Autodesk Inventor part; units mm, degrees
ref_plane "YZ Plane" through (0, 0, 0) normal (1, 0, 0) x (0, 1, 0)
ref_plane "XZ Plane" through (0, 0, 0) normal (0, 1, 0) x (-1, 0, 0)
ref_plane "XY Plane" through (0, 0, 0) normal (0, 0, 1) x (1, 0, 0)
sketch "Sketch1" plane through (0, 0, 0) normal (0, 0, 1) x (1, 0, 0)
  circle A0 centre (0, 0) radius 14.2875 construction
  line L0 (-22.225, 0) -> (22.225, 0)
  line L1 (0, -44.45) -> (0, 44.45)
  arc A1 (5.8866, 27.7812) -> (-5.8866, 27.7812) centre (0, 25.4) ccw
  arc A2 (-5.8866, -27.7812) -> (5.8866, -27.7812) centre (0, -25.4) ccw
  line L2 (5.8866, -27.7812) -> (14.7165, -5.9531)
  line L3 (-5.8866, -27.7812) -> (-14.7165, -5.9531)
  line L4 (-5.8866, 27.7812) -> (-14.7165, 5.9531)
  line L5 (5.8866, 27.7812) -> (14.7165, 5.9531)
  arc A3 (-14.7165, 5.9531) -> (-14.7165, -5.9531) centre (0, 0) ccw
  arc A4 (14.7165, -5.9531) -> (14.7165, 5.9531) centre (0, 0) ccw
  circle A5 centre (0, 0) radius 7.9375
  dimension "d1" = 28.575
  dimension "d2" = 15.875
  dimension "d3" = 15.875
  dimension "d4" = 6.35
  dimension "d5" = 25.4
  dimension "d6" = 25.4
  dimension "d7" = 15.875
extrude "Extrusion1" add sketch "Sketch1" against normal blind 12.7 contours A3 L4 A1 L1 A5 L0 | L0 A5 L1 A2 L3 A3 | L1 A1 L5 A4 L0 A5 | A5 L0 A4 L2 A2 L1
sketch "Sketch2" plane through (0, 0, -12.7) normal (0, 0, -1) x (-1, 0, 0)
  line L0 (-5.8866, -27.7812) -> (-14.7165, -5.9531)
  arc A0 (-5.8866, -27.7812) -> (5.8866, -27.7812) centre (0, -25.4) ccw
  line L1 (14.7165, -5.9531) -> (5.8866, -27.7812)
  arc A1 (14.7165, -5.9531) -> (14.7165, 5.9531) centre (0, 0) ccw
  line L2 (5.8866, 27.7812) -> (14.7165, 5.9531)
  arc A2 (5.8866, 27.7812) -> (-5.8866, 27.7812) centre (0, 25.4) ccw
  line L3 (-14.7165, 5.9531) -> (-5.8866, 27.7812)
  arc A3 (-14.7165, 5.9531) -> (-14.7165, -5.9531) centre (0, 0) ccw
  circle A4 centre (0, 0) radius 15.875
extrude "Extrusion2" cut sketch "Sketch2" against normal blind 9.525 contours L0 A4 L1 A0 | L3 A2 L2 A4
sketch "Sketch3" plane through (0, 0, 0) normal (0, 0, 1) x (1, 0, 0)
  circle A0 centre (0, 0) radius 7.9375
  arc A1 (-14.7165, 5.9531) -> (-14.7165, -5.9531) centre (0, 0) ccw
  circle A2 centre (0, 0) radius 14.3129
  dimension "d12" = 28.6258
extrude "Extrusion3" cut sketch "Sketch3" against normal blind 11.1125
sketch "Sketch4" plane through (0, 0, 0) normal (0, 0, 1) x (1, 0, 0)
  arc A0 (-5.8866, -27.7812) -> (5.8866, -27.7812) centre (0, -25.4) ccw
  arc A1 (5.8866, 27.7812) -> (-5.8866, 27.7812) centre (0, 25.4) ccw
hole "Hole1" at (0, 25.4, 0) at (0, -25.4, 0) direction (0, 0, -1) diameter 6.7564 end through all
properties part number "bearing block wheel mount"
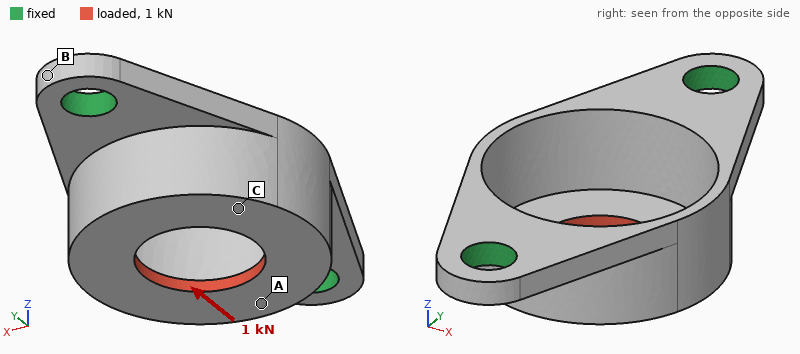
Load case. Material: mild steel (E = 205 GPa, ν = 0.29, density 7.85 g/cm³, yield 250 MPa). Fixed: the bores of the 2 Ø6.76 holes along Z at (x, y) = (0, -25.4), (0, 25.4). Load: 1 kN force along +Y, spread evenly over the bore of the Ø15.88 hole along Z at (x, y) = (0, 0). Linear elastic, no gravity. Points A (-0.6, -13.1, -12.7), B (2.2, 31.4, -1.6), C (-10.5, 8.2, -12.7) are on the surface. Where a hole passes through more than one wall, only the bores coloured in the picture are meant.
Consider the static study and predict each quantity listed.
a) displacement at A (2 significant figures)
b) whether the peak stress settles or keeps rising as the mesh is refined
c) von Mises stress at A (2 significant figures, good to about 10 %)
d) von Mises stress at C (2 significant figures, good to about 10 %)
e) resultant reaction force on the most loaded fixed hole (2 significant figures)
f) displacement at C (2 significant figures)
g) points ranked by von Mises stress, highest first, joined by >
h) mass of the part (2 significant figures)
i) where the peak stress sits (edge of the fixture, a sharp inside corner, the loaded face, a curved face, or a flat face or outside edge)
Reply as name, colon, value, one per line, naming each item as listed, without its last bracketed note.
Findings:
displacement at A: 7.3 µm
whether the peak stress settles or keeps rising as the mesh is refined: keeps rising
von Mises stress at A: 29 MPa
von Mises stress at C: 15 MPa
resultant reaction force on the most loaded fixed hole: 570 N
displacement at C: 6.3 µm
points ranked by von Mises stress, highest first, joined by >: A > C > B
mass of the part: 32 g
where the peak stress sits: edge of the fixture
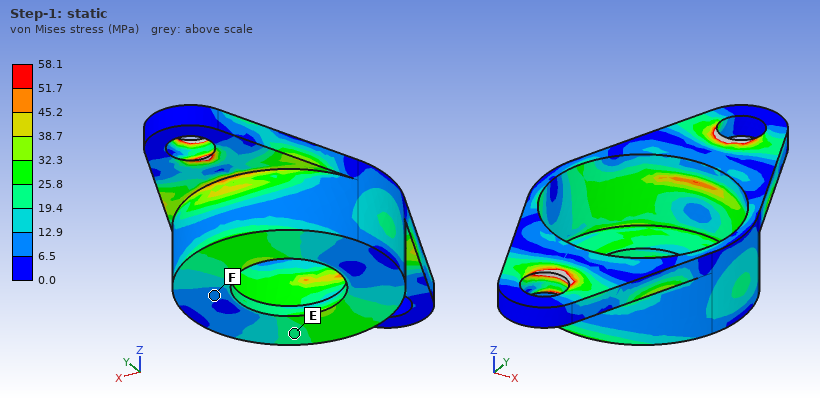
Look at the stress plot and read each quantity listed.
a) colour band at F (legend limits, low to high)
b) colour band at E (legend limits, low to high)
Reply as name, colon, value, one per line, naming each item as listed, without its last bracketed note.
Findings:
colour band at F: 6.5 to 12.9 MPa
colour band at E: 19.4 to 25.8 MPa
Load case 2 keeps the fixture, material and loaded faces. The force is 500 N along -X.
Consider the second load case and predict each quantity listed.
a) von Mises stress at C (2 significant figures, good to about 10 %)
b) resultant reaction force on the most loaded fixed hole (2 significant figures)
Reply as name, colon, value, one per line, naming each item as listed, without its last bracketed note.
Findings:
von Mises stress at C: 12 MPa
resultant reaction force on the most loaded fixed hole: 250 N
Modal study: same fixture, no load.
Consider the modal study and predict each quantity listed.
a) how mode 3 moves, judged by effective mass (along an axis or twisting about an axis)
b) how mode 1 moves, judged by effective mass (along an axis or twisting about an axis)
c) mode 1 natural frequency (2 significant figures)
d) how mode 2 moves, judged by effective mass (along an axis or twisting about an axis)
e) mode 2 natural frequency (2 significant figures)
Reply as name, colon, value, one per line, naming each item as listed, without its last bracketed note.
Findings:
how mode 3 moves, judged by effective mass: along Y
how mode 1 moves, judged by effective mass: along X
mode 1 natural frequency: 5100 Hz
how mode 2 moves, judged by effective mass: along Z
mode 2 natural frequency: 10 kHz
